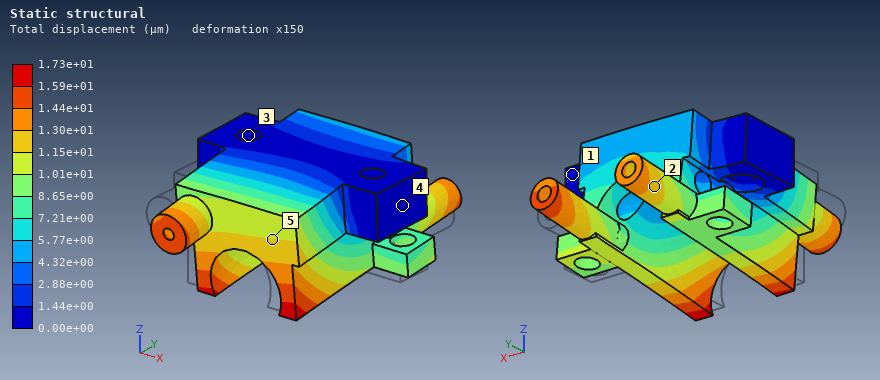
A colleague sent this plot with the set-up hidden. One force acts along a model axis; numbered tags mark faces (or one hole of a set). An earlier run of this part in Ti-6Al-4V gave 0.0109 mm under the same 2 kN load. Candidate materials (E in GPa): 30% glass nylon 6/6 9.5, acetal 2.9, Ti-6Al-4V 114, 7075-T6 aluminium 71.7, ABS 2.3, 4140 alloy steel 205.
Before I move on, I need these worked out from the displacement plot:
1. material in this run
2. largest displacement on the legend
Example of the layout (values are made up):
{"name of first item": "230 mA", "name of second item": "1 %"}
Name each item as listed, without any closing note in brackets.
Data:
{"material in this run": "7075-T6 aluminium", "largest displacement on the legend": "1.73e+01 µm"}
